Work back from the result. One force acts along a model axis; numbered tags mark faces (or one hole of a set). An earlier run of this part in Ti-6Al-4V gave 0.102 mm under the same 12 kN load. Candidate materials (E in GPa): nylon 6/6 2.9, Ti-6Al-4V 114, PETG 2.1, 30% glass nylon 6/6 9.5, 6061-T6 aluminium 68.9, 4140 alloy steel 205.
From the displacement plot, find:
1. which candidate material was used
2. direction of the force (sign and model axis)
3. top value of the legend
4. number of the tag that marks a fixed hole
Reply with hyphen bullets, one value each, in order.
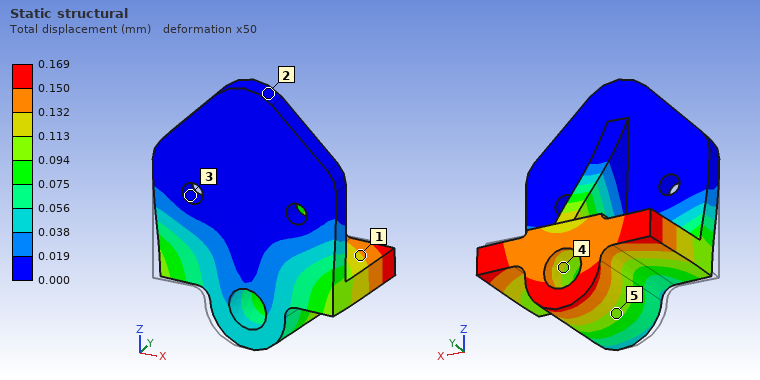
- 6061-T6 aluminium
- +X
- 0.169 mm
- 3
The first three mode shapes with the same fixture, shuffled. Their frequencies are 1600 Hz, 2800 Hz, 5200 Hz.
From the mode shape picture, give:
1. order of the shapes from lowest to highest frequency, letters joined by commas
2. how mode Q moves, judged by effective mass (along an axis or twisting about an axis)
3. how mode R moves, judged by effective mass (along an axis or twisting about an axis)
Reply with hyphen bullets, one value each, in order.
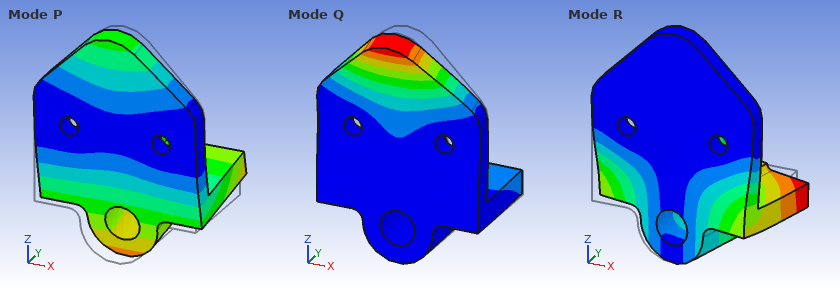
- P, R, Q
- along Y
- along X
